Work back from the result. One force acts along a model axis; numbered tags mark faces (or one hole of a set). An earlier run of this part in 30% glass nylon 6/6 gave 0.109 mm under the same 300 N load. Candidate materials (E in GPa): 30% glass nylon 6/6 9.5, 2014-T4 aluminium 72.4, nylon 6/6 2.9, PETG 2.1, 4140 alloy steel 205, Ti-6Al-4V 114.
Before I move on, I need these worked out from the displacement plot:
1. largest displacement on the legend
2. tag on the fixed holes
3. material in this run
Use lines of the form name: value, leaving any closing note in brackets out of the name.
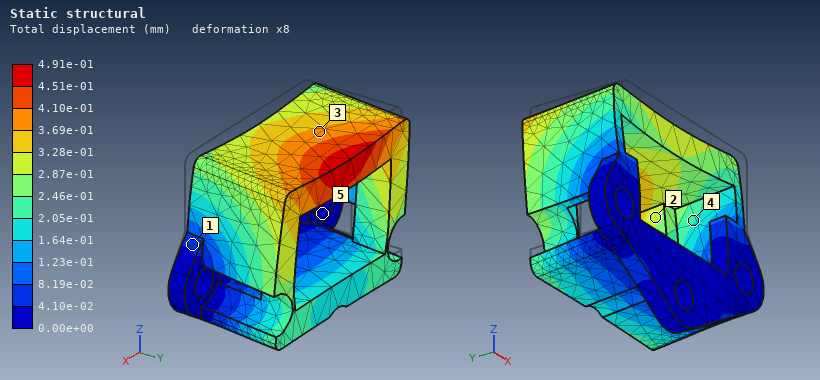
largest displacement on the legend: 4.91e-01 mm
tag on the fixed holes: 5
material in this run: PETG
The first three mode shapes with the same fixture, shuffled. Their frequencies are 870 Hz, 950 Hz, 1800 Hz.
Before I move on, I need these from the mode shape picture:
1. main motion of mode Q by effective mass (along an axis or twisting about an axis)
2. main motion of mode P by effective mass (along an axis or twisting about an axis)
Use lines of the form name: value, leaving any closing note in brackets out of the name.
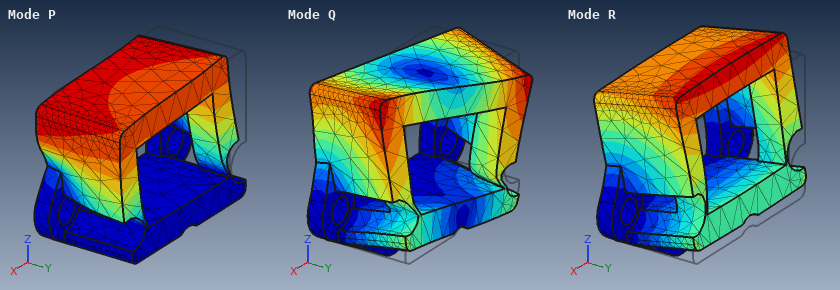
main motion of mode Q by effective mass: twisting about Z
main motion of mode P by effective mass: along X
